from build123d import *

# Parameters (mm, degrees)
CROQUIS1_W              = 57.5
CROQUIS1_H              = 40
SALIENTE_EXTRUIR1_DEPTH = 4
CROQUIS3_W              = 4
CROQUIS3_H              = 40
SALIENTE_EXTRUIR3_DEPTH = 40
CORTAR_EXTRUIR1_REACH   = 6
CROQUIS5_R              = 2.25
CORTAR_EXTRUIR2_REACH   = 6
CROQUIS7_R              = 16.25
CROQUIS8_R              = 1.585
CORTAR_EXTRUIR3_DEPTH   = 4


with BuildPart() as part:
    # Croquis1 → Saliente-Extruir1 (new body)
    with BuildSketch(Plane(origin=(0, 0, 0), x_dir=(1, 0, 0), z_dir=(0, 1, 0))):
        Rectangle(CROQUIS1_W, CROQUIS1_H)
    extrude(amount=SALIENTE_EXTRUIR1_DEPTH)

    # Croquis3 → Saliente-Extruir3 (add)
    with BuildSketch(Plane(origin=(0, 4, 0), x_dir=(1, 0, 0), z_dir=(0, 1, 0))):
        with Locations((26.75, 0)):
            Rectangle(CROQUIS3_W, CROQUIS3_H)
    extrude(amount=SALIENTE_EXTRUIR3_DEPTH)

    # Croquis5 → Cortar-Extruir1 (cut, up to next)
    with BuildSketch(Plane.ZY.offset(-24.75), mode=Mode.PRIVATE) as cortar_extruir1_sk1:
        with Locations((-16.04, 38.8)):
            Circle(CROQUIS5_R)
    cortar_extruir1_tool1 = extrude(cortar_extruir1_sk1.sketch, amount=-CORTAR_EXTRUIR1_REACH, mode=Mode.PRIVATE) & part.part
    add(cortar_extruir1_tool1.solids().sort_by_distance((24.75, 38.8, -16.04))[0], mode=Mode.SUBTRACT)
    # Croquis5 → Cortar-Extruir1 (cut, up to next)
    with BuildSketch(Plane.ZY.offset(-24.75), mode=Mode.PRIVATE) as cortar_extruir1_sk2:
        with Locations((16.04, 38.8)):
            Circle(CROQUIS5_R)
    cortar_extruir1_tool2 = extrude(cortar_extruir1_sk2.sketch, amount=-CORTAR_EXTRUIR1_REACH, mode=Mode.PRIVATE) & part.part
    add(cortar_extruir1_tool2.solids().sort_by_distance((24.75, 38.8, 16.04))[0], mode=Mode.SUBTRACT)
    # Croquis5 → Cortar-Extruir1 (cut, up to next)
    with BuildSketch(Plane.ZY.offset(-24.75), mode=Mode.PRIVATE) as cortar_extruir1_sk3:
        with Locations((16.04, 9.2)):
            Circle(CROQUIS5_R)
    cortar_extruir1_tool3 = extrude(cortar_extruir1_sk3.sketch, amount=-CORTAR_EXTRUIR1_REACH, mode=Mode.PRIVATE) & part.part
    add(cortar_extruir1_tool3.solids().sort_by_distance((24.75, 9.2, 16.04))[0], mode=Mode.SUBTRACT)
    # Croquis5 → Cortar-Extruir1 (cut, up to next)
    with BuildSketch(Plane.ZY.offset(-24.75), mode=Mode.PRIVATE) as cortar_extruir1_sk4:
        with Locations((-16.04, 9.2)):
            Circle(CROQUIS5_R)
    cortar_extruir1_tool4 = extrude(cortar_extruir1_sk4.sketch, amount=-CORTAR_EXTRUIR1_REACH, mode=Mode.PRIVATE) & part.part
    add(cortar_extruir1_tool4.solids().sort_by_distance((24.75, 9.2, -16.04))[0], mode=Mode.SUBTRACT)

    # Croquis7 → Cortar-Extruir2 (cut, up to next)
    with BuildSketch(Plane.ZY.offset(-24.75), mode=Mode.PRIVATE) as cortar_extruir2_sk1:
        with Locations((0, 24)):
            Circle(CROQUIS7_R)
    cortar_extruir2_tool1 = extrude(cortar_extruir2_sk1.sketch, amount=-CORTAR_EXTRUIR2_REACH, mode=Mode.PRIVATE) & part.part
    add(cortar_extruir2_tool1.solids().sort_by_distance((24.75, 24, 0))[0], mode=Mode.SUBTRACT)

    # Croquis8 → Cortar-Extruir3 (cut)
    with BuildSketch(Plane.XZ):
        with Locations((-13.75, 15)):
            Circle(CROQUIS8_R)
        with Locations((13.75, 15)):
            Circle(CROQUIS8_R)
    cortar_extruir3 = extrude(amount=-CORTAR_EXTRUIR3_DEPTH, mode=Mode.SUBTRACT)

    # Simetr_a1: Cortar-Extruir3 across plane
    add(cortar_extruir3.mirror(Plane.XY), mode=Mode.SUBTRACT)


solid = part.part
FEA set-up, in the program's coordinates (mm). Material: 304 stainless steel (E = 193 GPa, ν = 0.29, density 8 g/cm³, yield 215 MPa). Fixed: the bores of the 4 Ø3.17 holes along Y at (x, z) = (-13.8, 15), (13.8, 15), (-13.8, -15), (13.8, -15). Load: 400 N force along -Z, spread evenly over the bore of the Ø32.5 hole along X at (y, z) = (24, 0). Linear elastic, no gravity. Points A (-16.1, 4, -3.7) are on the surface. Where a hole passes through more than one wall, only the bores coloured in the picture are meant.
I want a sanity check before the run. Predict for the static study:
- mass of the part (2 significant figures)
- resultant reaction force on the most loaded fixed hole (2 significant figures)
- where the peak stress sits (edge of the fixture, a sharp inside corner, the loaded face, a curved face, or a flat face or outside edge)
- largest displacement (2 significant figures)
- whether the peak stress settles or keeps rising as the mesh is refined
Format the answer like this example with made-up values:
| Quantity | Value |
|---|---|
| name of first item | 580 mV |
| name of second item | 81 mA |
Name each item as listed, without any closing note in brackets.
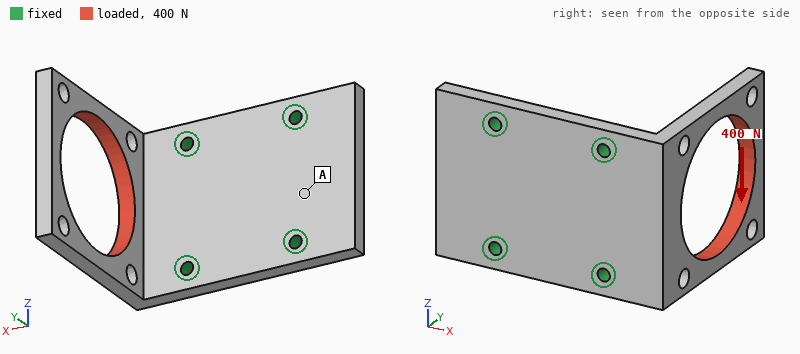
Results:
| Quantity | Value |
|---|---|
| mass of the part | 95 g |
| resultant reaction force on the most loaded fixed hole | 380 N |
| where the peak stress sits | edge of the fixture |
| largest displacement | 51 µm |
| whether the peak stress settles or keeps rising as the mesh is refined | keeps rising |
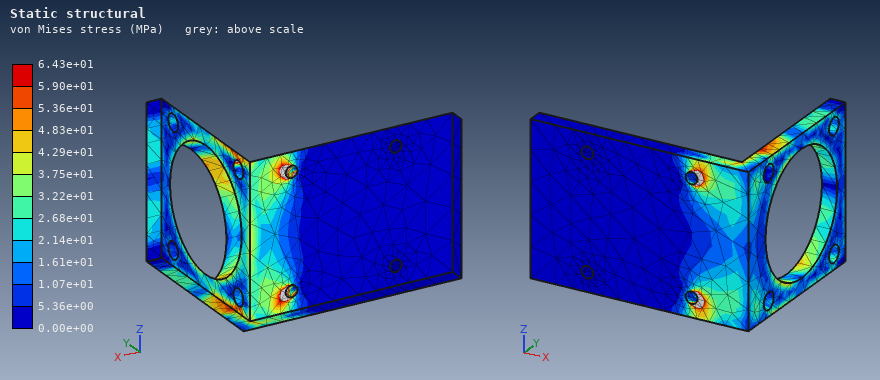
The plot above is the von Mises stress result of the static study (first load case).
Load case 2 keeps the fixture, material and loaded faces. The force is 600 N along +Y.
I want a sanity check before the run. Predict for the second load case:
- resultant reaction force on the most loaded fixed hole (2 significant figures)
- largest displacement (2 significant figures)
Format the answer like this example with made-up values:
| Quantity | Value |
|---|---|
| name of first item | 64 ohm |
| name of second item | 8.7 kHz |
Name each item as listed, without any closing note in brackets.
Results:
| Quantity | Value |
|---|---|
| resultant reaction force on the most loaded fixed hole | 340 N |
| largest displacement | 64 µm |
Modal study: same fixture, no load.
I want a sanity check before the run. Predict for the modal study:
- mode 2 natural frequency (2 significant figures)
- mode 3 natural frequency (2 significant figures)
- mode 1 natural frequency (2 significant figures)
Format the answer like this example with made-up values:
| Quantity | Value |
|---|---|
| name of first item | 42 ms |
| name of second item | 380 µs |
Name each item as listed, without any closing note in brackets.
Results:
| Quantity | Value |
|---|---|
| mode 2 natural frequency | 2700 Hz |
| mode 3 natural frequency | 3500 Hz |
| mode 1 natural frequency | 1200 Hz |
